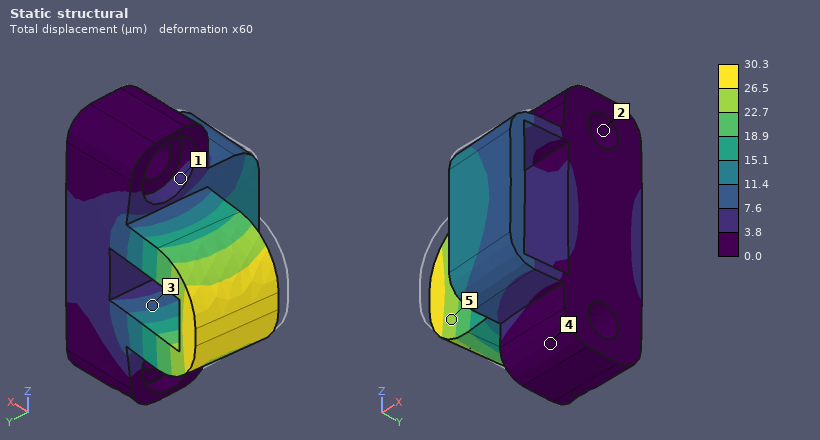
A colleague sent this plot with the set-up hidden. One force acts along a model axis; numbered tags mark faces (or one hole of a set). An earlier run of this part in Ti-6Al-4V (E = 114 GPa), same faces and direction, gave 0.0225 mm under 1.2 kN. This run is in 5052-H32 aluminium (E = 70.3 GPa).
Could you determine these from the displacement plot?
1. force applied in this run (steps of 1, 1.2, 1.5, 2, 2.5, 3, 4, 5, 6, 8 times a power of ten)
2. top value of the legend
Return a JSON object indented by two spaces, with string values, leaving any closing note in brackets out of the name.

{
  "force applied in this run": "1 kN",
  "top value of the legend": "30.3 µm"
}
